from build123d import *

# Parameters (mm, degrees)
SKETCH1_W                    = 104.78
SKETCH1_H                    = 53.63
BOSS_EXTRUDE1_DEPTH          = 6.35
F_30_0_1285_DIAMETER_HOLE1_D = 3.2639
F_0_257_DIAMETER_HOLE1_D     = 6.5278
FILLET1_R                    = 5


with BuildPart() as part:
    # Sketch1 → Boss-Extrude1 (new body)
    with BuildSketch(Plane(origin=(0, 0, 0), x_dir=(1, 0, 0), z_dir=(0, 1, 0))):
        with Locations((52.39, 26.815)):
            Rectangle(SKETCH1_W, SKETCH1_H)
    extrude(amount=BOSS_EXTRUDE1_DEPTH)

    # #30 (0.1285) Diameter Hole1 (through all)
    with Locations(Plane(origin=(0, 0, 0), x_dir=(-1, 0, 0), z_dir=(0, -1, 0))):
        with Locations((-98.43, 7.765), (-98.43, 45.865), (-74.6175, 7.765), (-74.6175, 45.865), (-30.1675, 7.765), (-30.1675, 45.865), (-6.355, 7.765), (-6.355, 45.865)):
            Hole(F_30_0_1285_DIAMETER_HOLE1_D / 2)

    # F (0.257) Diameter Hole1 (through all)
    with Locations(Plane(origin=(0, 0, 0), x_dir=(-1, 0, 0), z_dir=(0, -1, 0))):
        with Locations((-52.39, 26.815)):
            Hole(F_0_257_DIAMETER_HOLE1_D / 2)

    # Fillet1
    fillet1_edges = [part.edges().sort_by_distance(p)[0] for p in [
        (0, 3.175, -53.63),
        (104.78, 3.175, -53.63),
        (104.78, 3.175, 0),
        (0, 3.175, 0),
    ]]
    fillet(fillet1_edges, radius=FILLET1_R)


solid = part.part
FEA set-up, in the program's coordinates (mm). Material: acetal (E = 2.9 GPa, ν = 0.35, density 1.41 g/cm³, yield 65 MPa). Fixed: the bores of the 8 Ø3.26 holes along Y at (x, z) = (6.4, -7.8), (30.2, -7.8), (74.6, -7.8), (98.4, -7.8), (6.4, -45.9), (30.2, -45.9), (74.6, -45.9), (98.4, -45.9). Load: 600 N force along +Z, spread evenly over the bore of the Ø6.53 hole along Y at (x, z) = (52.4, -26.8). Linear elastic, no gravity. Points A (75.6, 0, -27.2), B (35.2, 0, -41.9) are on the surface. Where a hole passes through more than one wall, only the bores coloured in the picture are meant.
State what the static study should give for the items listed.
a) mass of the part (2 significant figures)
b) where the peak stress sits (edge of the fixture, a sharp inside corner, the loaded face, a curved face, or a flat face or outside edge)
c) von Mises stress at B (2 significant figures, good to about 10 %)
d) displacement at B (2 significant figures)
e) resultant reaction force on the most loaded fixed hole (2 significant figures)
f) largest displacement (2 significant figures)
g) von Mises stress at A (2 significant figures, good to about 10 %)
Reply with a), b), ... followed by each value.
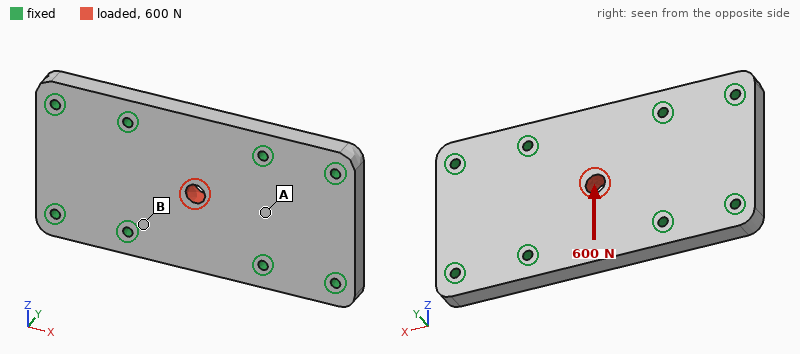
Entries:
a) 49 g
b) the loaded face
c) 2.3 MPa
d) 6.4 µm
e) 160 N
f) 30 µm
g) 0.70 MPa
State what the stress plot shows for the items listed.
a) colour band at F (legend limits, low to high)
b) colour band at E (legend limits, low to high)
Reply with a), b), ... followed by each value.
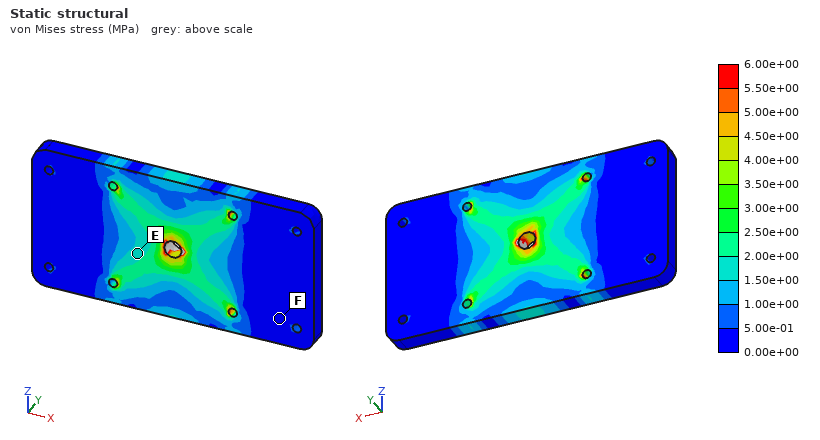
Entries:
a) 0.00e+00 to 5.00e-01 MPa
b) 1.50e+00 to 2.00e+00 MPa
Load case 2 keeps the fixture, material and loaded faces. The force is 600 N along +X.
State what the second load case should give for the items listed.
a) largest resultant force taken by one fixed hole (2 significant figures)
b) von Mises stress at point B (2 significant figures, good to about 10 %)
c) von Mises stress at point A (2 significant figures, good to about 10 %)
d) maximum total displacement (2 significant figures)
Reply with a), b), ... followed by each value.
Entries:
a) 120 N
b) 1.7 MPa
c) 0.87 MPa
d) 22 µm
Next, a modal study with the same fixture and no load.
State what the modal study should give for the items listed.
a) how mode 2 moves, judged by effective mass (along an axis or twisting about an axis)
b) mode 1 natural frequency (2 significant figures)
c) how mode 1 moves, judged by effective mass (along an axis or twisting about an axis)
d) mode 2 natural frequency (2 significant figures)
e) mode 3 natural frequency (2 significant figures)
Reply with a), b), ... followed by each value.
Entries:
a) twisting about X
b) 3300 Hz
c) along Y
d) 4500 Hz
e) 4900 Hz
